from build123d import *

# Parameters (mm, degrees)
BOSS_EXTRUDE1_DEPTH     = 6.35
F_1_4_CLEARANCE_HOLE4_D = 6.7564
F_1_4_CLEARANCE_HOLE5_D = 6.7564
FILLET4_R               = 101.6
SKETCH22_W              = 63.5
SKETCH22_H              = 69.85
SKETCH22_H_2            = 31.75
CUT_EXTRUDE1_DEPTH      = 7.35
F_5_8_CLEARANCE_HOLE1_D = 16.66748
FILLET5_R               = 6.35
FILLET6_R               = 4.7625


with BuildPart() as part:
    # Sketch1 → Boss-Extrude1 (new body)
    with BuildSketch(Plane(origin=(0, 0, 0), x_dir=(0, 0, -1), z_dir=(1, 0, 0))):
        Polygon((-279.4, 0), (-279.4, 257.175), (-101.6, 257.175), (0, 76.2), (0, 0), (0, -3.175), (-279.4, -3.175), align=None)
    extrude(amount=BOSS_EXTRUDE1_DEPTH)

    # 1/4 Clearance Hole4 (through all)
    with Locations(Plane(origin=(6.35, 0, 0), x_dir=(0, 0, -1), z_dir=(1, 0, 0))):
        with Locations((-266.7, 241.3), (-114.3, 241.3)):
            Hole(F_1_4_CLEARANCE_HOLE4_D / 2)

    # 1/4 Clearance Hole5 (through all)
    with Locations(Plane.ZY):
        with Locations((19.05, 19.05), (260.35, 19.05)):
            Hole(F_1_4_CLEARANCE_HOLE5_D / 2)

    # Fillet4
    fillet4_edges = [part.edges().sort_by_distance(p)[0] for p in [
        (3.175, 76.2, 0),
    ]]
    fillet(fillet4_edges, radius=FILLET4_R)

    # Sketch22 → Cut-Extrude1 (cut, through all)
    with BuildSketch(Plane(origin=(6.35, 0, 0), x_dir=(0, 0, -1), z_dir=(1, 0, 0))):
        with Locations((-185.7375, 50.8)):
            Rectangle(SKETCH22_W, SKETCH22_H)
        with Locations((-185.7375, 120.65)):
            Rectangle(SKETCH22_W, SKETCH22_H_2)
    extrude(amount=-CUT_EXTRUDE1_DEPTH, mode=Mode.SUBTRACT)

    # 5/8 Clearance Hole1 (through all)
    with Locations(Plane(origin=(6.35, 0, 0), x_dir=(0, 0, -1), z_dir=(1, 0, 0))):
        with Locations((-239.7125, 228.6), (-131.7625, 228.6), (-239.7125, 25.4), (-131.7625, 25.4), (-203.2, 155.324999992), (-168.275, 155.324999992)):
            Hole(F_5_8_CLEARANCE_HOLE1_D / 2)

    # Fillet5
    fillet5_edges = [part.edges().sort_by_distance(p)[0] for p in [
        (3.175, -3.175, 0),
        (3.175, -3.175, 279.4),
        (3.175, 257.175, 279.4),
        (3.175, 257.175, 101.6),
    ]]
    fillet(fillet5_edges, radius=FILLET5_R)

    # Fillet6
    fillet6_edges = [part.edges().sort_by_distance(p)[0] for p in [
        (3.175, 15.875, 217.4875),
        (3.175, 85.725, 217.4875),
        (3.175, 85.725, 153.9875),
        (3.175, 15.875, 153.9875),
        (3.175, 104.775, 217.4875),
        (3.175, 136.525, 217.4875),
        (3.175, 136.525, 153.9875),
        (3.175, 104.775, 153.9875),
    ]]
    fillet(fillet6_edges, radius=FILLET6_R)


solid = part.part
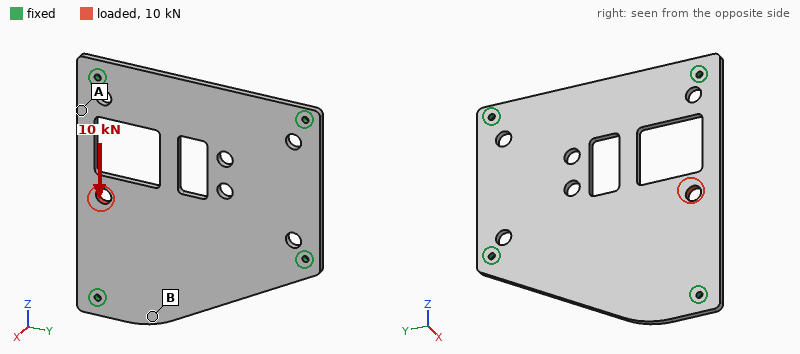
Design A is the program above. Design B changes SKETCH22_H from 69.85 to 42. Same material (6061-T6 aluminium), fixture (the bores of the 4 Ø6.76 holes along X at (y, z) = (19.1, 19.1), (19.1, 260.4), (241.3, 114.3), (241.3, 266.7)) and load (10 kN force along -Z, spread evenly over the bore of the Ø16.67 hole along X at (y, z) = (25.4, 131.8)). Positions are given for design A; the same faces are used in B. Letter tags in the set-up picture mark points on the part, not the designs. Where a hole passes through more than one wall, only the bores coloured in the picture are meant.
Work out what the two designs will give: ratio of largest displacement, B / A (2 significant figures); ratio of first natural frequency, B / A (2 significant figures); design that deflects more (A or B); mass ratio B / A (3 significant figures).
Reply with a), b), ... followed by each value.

a) 0.80
b) 1.0
c) A
d) 1.03
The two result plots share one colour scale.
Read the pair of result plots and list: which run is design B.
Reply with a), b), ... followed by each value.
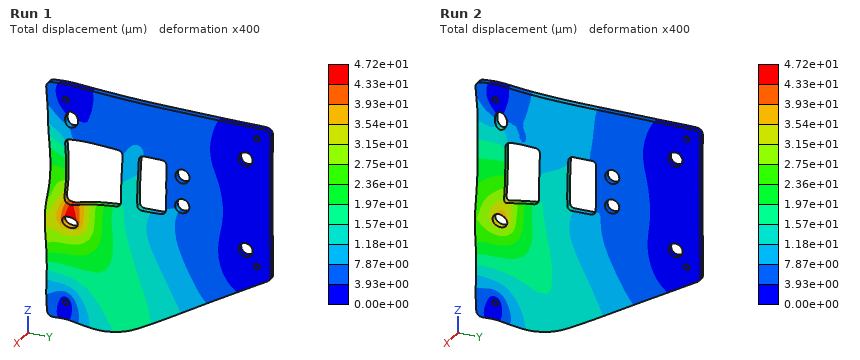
a) Run 2
